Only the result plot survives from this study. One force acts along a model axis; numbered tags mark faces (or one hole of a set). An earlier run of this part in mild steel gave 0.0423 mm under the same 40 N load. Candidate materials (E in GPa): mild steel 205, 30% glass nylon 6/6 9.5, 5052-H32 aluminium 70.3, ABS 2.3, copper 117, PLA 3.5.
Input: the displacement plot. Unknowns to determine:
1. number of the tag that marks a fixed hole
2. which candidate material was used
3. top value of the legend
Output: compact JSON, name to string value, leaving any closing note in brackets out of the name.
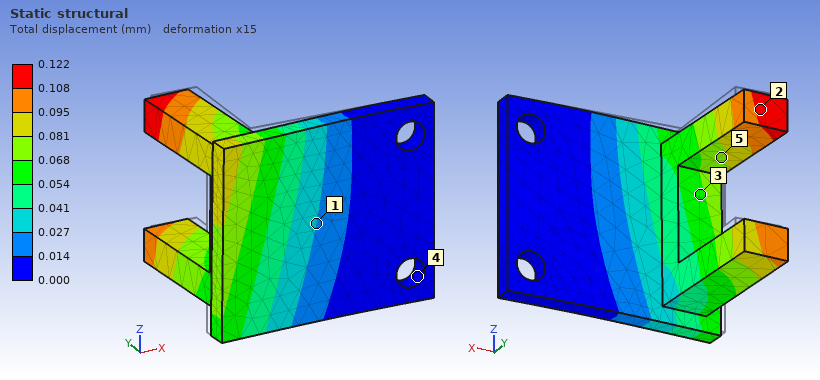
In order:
{"number of the tag that marks a fixed hole": "4", "which candidate material was used": "5052-H32 aluminium", "top value of the legend": "0.122 mm"}
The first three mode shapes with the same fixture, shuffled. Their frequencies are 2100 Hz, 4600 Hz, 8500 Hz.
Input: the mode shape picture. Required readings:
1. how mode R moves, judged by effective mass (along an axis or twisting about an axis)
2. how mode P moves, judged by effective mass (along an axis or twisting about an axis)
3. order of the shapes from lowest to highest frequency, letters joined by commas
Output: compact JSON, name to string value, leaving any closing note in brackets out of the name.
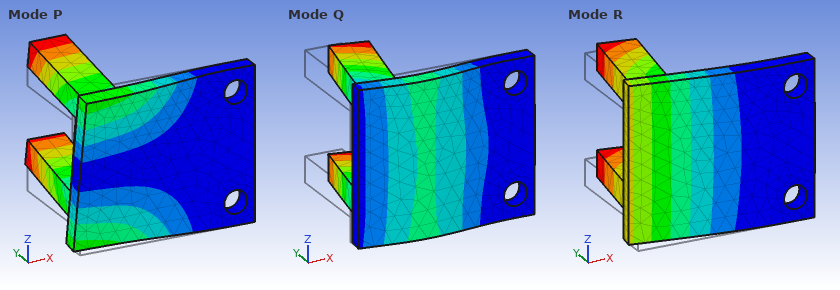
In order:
{"how mode R moves, judged by effective mass": "along Y", "how mode P moves, judged by effective mass": "along Z", "order of the shapes from lowest to highest frequency, letters joined by commas": "R, P, Q"}
